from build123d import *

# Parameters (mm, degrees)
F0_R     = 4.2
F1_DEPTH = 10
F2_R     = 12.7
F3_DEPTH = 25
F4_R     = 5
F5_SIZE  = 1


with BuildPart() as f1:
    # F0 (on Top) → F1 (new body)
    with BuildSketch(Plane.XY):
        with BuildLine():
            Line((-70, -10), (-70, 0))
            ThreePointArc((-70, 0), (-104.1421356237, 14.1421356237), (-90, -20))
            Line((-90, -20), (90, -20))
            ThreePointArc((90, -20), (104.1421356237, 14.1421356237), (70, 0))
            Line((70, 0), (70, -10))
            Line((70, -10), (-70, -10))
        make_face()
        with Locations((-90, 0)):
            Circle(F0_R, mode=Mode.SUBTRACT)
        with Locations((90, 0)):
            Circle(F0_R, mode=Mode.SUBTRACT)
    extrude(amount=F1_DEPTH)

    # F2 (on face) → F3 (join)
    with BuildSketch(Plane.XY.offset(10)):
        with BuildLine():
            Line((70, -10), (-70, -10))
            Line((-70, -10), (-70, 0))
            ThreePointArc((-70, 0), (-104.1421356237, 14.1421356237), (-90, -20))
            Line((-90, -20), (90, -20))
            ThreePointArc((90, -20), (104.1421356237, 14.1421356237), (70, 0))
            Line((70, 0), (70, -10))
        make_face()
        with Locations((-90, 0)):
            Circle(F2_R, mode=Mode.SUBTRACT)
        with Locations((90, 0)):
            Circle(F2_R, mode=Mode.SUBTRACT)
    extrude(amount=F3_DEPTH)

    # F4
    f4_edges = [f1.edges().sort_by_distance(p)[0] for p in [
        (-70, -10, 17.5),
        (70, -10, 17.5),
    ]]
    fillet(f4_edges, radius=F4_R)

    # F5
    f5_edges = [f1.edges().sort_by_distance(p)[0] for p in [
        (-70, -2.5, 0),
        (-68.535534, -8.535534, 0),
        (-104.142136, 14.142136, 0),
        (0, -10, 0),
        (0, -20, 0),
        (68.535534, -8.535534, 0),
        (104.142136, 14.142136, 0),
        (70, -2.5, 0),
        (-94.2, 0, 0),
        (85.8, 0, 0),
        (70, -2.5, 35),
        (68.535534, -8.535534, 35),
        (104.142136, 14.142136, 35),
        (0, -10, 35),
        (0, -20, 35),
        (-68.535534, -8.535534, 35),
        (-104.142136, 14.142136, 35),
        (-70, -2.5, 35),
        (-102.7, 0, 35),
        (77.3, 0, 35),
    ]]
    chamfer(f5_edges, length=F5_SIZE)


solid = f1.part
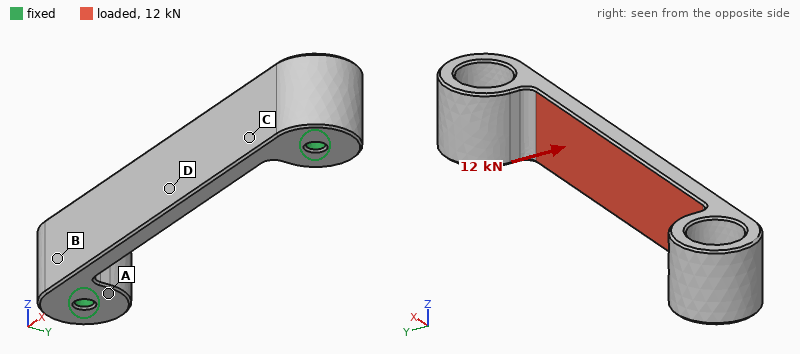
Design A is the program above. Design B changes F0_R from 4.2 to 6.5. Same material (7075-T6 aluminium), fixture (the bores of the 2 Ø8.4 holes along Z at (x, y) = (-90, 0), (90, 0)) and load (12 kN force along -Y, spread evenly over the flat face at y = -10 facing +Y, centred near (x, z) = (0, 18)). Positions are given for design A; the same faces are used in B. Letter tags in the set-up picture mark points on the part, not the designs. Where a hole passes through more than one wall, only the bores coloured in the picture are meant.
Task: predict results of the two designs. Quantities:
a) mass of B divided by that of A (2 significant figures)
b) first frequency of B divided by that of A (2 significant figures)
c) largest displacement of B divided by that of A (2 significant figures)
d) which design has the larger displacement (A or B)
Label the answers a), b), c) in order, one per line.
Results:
a) 0.99
b) 1.1
c) 0.89
d) A
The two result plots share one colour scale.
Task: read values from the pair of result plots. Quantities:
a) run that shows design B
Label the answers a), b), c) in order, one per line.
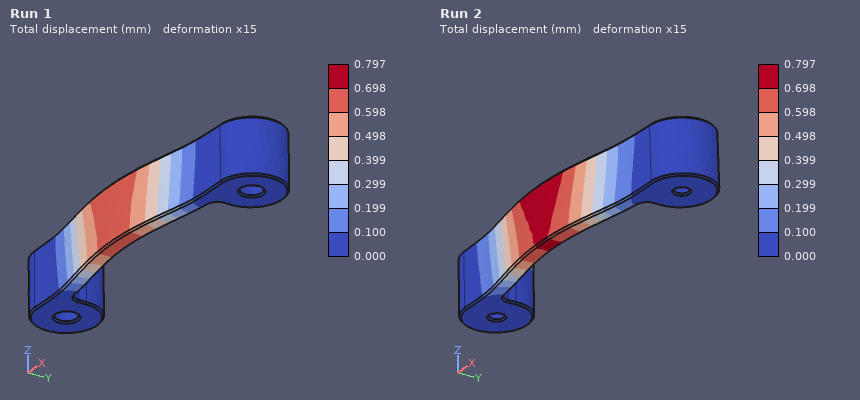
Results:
a) Run 1
